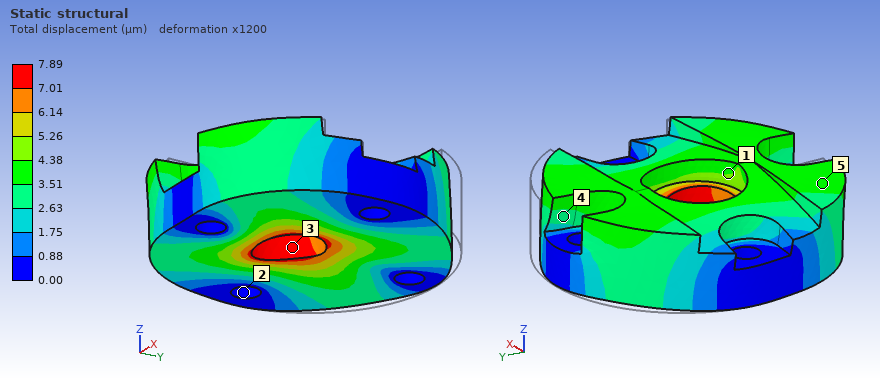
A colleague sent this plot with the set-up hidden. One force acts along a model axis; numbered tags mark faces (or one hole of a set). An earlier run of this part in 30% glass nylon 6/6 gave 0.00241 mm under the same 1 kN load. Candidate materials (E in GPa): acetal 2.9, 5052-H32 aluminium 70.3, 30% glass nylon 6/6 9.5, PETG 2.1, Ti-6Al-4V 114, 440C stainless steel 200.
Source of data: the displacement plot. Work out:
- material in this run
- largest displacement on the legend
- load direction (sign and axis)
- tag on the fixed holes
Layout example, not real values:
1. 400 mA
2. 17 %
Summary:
1. acetal
2. 7.89 µm
3. -Y
4. 2
